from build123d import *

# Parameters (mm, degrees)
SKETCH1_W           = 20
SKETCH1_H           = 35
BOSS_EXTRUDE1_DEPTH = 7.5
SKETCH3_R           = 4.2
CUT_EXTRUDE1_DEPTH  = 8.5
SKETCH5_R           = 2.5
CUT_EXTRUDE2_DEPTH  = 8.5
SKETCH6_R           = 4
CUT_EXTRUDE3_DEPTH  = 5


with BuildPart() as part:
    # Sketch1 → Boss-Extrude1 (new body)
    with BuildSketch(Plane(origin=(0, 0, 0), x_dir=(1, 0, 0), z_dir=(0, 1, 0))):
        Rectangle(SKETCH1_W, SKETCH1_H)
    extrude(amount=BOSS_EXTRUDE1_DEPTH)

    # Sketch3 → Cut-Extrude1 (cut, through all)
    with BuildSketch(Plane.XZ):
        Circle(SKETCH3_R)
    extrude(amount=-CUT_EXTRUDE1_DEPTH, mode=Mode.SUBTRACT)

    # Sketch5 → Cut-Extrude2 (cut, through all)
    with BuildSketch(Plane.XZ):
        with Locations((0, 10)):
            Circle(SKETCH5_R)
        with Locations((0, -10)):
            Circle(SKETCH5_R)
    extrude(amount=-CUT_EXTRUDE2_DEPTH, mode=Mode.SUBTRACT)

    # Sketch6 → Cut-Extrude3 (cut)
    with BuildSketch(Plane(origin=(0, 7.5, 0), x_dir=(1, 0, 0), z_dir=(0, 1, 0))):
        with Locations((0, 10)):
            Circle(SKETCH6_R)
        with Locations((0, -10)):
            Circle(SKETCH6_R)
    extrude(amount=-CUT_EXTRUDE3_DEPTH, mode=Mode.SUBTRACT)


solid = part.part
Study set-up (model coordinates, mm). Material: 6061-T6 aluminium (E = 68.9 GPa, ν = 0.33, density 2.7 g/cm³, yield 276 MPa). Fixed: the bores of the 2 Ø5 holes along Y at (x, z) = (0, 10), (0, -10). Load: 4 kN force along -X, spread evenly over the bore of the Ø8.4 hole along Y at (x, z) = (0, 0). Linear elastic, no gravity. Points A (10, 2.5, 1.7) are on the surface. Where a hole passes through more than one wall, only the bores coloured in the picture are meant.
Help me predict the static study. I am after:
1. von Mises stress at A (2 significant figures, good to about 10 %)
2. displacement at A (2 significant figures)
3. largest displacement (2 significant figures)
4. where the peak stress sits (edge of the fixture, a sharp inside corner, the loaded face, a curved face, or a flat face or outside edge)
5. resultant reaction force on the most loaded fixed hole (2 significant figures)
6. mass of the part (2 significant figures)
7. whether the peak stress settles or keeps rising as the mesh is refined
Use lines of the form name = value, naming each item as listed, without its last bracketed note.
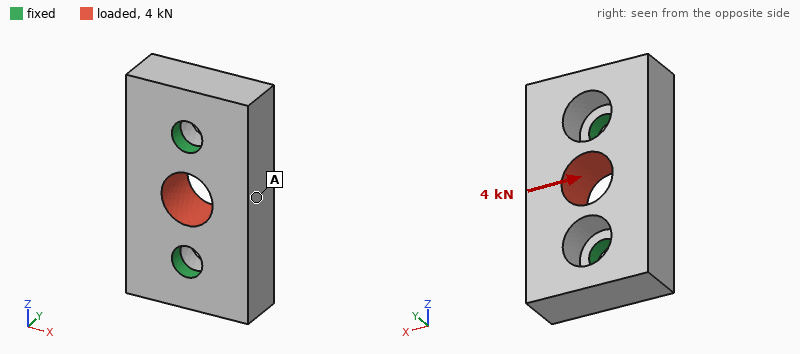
von Mises stress at A = 44 MPa
displacement at A = 26 µm
largest displacement = 35 µm
where the peak stress sits = edge of the fixture
resultant reaction force on the most loaded fixed hole = 2.0 kN
mass of the part = 11 g
whether the peak stress settles or keeps rising as the mesh is refined = keeps rising
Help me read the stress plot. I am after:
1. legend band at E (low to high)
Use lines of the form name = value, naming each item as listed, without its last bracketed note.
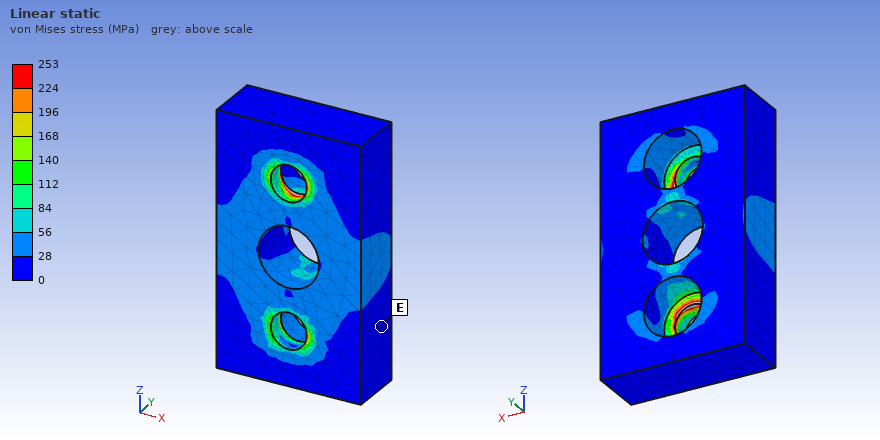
legend band at E = 0 to 28 MPa
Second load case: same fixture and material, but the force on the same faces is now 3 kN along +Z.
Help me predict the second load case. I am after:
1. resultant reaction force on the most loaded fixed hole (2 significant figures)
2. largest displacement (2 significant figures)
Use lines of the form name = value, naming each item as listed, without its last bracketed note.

resultant reaction force on the most loaded fixed hole = 1.5 kN
largest displacement = 8.1 µm
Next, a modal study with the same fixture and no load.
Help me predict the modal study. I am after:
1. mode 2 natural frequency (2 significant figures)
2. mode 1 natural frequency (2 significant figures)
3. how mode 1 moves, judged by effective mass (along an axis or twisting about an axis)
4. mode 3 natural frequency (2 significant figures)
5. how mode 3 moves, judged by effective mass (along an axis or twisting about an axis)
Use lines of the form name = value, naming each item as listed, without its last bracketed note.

mode 2 natural frequency = 25 kHz
mode 1 natural frequency = 15 kHz
how mode 1 moves, judged by effective mass = along X
mode 3 natural frequency = 31 kHz
how mode 3 moves, judged by effective mass = along Z
